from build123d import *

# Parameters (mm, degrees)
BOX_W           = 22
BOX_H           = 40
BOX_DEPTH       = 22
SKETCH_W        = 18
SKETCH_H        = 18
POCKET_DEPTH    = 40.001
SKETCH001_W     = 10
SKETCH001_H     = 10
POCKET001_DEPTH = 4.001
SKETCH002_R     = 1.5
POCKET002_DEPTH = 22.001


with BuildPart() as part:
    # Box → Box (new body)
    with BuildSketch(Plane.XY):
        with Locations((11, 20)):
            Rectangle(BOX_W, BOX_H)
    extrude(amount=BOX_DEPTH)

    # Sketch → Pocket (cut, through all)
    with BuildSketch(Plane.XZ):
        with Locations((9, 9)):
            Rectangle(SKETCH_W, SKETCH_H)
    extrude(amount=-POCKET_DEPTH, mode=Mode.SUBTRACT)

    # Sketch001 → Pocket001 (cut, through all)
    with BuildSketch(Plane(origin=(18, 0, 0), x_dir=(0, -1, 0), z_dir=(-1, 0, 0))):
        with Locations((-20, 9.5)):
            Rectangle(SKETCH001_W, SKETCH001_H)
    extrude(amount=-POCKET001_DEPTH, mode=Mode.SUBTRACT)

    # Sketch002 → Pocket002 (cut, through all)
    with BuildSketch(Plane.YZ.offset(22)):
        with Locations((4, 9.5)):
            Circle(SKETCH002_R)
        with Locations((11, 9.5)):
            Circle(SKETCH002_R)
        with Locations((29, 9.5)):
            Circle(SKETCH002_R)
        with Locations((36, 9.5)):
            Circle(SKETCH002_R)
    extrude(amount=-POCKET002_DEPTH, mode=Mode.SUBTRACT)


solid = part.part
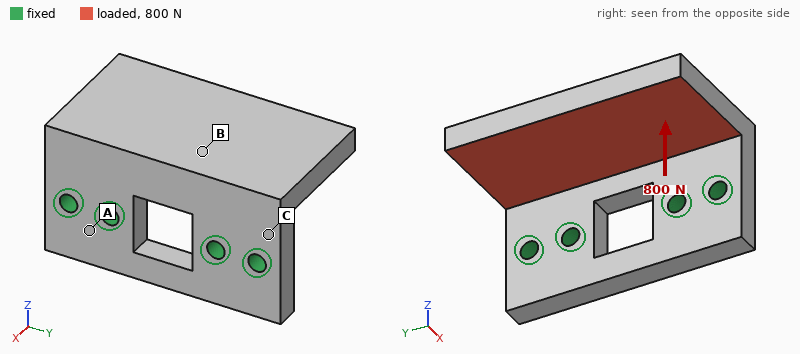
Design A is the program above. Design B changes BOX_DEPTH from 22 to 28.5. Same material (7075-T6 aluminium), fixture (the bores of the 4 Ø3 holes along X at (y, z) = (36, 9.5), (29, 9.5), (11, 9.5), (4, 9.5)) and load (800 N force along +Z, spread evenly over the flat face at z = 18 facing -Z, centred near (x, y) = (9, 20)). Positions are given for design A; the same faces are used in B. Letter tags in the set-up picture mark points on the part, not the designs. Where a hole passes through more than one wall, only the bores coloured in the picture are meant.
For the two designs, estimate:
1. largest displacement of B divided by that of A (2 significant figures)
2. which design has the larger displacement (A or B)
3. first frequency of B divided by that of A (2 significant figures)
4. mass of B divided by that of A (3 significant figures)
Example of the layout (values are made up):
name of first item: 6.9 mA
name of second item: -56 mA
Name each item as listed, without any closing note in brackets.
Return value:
largest displacement of B divided by that of A: 0.89
which design has the larger displacement: A
first frequency of B divided by that of A: 0.58
mass of B divided by that of A: 1.97
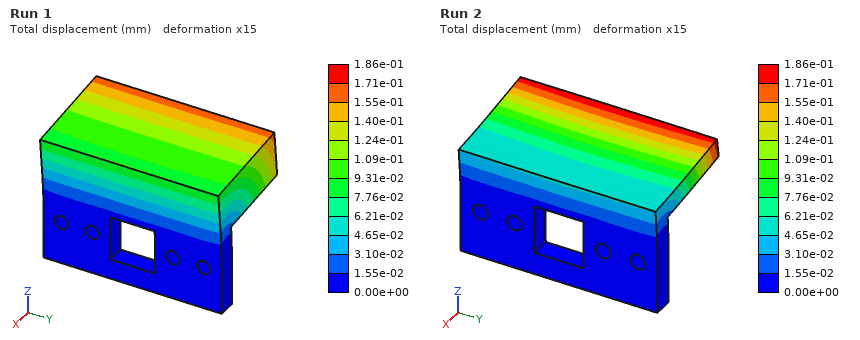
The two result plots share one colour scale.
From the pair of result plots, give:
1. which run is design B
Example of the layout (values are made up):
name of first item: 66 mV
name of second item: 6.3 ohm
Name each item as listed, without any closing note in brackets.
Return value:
which run is design B: Run 1
